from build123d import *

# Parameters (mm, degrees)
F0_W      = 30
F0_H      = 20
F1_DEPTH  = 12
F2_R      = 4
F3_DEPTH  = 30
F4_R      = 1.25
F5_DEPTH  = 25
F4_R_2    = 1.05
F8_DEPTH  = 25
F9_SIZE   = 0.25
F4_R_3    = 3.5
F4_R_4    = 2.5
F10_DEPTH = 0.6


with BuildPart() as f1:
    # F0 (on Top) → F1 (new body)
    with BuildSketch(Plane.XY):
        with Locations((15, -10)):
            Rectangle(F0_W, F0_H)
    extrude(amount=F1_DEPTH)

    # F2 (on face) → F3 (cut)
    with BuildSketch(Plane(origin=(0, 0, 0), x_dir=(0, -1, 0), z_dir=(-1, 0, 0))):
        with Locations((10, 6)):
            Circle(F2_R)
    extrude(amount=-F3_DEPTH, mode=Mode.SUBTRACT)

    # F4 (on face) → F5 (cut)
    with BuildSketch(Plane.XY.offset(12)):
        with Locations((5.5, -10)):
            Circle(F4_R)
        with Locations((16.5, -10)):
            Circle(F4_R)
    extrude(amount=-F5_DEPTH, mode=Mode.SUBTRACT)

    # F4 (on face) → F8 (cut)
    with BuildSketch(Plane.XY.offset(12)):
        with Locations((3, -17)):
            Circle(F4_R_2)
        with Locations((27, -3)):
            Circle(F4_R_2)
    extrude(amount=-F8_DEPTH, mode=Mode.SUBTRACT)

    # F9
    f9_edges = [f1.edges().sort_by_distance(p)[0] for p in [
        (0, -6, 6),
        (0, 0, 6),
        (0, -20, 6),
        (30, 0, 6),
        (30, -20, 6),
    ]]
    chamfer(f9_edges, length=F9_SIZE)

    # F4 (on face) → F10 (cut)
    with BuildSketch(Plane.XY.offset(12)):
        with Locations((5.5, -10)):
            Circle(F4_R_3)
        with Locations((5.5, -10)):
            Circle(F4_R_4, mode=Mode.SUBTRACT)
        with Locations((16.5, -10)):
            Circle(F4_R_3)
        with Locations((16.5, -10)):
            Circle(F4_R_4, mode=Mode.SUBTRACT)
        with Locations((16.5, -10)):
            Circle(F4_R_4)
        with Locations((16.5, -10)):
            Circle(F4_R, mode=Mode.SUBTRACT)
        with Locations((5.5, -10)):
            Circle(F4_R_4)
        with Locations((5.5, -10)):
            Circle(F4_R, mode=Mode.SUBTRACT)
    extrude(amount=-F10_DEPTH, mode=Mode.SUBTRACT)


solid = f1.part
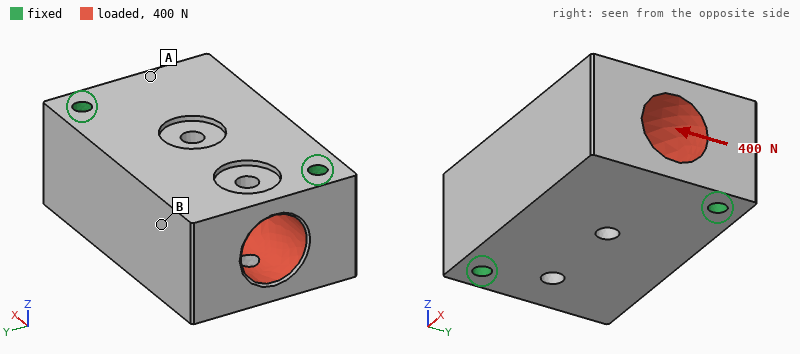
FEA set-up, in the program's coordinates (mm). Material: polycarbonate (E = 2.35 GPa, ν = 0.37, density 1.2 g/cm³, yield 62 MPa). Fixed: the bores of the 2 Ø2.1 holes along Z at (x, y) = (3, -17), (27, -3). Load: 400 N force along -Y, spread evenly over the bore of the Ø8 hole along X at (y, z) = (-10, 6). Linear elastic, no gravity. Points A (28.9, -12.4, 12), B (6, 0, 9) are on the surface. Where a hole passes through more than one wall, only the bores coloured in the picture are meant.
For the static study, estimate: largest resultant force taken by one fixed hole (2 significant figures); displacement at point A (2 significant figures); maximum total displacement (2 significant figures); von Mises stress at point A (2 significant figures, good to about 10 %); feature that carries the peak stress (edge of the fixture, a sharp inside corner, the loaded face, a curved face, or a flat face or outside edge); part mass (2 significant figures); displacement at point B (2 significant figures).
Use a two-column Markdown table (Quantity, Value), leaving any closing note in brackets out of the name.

| Quantity | Value |
|---|---|
| largest resultant force taken by one fixed hole | 210 N |
| displacement at point A | 12 µm |
| maximum total displacement | 23 µm |
| von Mises stress at point A | 2.0 MPa |
| feature that carries the peak stress | the loaded face |
| part mass | 6.6 g |
| displacement at point B | 20 µm |
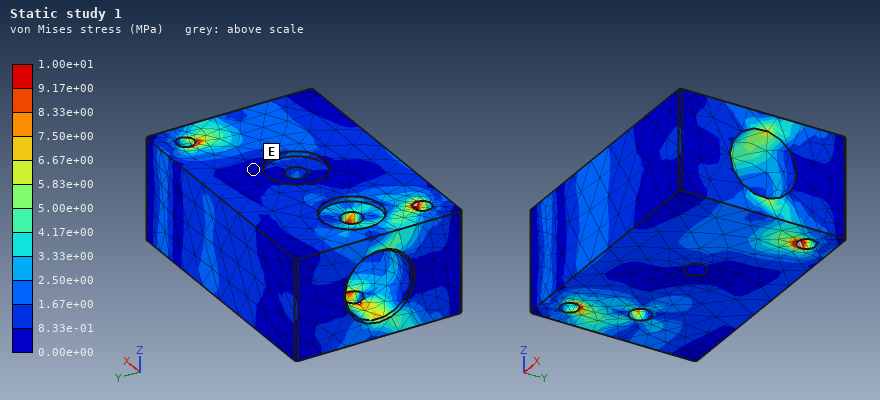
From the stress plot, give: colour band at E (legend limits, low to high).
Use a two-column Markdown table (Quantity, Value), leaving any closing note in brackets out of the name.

| Quantity | Value |
|---|---|
| colour band at E | 0.00e+00 to 8.33e-01 MPa |
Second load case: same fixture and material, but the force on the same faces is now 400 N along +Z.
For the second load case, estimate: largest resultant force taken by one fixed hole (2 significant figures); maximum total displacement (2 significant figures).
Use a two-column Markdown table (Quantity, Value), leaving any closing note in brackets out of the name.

| Quantity | Value |
|---|---|
| largest resultant force taken by one fixed hole | 200 N |
| maximum total displacement | 57 µm |
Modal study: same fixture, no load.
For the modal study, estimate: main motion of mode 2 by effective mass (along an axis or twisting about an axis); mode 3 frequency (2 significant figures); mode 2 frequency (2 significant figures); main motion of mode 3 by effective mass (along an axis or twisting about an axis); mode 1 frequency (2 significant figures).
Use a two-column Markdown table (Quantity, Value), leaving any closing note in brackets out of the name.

| Quantity | Value |
|---|---|
| main motion of mode 2 by effective mass | along Z |
| mode 3 frequency | 8900 Hz |
| mode 2 frequency | 6000 Hz |
| main motion of mode 3 by effective mass | along Y |
| mode 1 frequency | 4900 Hz |
